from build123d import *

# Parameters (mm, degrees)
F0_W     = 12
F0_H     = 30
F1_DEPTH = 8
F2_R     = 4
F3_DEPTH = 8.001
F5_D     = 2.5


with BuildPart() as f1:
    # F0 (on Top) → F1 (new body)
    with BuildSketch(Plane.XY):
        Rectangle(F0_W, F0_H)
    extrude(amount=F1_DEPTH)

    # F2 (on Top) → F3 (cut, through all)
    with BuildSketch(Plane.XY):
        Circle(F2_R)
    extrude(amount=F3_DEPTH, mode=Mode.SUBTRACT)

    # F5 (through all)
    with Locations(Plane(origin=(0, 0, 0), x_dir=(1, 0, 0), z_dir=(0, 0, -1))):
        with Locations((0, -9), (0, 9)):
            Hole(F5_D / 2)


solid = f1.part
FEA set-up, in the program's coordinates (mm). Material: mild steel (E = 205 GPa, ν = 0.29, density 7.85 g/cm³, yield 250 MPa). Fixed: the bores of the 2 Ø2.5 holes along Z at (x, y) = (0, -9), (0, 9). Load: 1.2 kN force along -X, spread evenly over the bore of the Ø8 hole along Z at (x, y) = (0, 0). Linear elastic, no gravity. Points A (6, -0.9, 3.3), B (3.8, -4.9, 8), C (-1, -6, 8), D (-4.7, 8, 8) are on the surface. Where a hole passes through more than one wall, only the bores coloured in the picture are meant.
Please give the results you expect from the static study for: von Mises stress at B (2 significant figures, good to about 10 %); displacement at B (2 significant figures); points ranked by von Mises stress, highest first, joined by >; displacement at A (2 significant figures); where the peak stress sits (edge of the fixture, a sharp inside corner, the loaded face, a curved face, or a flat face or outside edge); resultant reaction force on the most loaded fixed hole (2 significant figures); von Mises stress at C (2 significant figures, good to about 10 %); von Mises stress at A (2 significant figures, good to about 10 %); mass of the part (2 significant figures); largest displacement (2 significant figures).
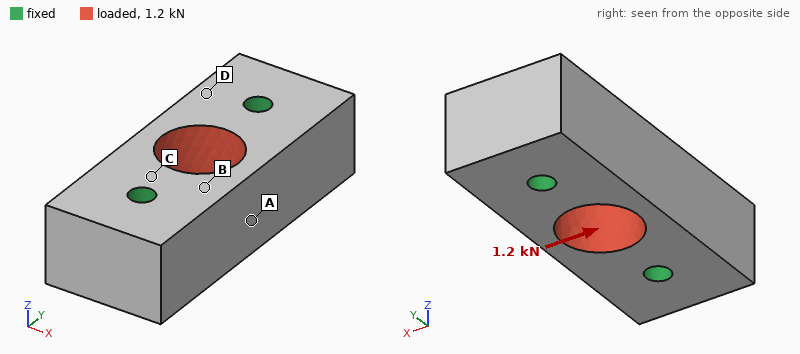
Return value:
12 MPa
0.59 µm
A > C > B > D
1.1 µm
edge of the fixture
600 N
18 MPa
27 MPa
19 g
1.3 µm
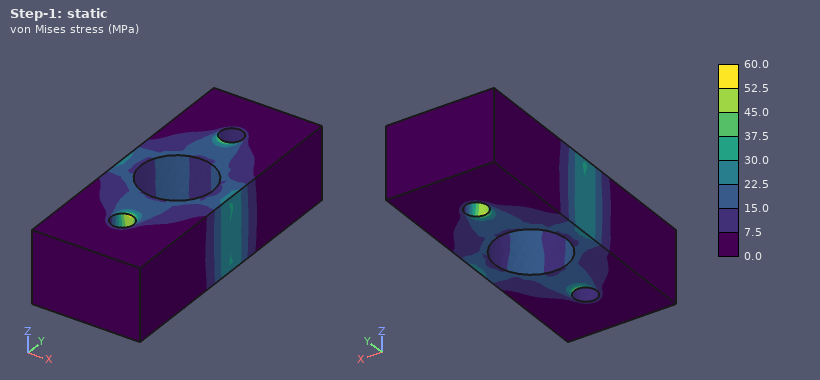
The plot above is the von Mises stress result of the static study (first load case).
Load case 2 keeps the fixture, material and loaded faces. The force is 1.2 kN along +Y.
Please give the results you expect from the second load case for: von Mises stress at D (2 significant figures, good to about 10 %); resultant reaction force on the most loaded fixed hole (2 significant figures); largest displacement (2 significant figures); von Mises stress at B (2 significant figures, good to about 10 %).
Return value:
3.5 MPa
600 N
0.42 µm
7.3 MPa
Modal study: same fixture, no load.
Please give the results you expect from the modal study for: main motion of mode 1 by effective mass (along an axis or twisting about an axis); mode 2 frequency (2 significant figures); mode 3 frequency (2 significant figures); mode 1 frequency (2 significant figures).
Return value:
twisting about Z
64 kHz
66 kHz
53 kHz
